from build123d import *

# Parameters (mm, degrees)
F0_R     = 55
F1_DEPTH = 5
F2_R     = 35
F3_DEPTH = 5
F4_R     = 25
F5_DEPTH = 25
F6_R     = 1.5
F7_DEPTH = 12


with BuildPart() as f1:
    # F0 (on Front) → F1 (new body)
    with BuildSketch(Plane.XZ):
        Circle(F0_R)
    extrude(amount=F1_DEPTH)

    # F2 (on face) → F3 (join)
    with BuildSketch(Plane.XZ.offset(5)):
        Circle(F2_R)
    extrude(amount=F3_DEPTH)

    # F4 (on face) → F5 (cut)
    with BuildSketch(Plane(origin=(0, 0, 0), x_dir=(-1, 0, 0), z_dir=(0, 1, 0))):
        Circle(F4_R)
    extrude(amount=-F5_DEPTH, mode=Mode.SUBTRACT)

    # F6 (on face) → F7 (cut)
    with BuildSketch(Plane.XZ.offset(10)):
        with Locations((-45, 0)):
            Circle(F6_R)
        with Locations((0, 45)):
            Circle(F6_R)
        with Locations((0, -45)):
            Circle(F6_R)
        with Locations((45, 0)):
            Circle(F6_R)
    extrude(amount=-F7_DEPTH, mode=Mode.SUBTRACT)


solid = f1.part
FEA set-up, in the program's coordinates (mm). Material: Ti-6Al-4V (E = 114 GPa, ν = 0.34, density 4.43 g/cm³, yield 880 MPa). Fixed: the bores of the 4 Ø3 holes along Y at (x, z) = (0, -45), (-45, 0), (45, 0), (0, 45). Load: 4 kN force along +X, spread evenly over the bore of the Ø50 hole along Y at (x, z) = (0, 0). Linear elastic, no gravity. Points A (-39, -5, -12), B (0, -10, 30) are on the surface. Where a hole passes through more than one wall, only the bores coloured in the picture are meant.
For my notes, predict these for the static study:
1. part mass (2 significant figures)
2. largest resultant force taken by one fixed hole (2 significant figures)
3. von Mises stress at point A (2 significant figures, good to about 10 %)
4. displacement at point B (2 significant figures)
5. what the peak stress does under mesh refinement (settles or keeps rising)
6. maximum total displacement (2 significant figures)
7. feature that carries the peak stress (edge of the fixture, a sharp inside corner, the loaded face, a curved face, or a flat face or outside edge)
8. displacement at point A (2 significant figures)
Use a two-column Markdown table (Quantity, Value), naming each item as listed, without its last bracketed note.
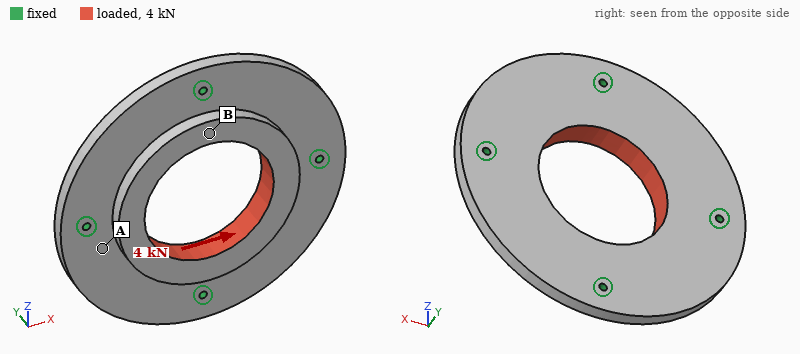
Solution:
| Quantity | Value |
|---|---|
| part mass | 210 g |
| largest resultant force taken by one fixed hole | 1.0 kN |
| von Mises stress at point A | 7.4 MPa |
| displacement at point B | 2.4 µm |
| what the peak stress does under mesh refinement | keeps rising |
| maximum total displacement | 3.4 µm |
| feature that carries the peak stress | edge of the fixture |
| displacement at point A | 1.8 µm |
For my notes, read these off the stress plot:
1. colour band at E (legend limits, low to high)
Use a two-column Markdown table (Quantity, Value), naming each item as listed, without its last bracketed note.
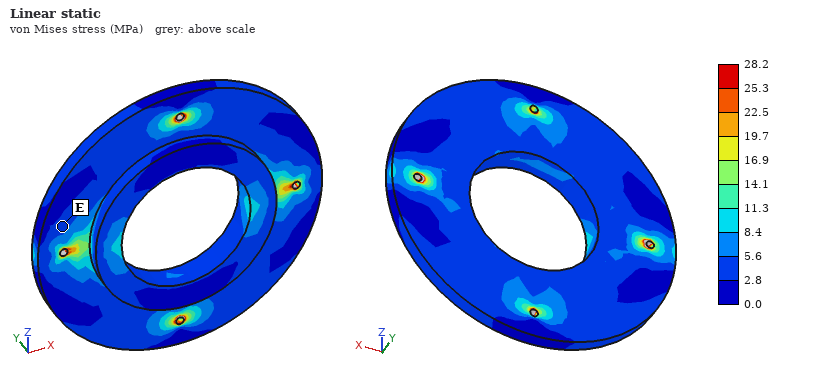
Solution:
| Quantity | Value |
|---|---|
| colour band at E | 2.8 to 5.6 MPa |
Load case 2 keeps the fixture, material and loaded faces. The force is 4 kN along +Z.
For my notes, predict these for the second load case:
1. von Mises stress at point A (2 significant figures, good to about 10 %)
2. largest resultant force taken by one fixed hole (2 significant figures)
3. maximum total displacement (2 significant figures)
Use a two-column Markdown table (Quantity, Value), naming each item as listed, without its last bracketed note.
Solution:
| Quantity | Value |
|---|---|
| von Mises stress at point A | 5.5 MPa |
| largest resultant force taken by one fixed hole | 1.0 kN |
| maximum total displacement | 3.4 µm |
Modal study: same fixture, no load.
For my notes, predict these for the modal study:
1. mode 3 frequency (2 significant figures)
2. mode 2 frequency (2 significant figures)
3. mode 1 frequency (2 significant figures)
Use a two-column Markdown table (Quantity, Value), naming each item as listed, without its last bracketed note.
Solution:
| Quantity | Value |
|---|---|
| mode 3 frequency | 5300 Hz |
| mode 2 frequency | 5300 Hz |
| mode 1 frequency | 4500 Hz |
